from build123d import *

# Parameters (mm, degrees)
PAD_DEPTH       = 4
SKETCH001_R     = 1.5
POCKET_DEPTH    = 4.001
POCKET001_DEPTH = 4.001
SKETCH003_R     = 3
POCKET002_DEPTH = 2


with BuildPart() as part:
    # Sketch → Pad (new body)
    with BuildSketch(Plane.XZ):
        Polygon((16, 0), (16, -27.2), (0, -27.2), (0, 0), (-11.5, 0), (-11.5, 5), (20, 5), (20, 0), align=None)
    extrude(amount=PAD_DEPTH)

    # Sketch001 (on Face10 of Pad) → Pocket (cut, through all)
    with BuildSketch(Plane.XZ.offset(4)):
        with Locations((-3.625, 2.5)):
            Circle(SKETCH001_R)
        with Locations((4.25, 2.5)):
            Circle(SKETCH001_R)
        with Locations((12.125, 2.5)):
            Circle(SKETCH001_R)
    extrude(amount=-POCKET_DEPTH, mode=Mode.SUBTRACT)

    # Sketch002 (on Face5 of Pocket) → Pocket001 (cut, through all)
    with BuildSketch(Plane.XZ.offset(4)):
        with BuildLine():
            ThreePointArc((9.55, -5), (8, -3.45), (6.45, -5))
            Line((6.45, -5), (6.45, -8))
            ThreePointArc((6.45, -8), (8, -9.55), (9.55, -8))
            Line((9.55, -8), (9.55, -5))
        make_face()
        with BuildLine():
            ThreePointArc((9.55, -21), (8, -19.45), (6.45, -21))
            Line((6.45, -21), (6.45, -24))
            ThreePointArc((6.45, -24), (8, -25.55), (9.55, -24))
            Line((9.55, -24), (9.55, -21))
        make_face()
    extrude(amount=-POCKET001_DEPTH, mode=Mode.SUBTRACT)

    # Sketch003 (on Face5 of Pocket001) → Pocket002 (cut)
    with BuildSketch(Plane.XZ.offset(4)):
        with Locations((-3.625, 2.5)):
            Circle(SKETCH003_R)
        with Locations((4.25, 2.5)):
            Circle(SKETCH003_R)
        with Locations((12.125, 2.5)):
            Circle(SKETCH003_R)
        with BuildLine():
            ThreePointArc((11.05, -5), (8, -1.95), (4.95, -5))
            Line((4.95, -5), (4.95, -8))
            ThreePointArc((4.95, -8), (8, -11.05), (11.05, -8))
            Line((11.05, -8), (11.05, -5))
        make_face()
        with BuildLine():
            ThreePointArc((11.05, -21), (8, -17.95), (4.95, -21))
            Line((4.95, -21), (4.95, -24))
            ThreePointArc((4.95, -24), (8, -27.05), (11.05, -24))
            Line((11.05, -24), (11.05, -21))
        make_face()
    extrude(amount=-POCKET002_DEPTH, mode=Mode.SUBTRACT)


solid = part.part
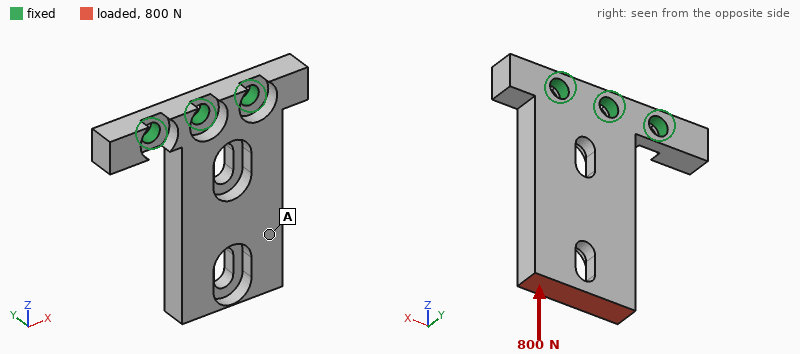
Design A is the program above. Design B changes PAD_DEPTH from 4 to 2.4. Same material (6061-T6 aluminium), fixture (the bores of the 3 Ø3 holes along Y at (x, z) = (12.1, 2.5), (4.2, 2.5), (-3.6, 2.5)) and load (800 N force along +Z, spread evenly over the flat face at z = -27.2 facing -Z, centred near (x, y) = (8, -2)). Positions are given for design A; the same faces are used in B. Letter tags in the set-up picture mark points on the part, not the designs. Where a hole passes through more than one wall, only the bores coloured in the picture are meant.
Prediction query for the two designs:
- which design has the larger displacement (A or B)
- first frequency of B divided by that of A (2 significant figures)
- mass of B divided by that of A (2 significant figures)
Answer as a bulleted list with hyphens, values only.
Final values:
- A
- 0.76
- 0.65
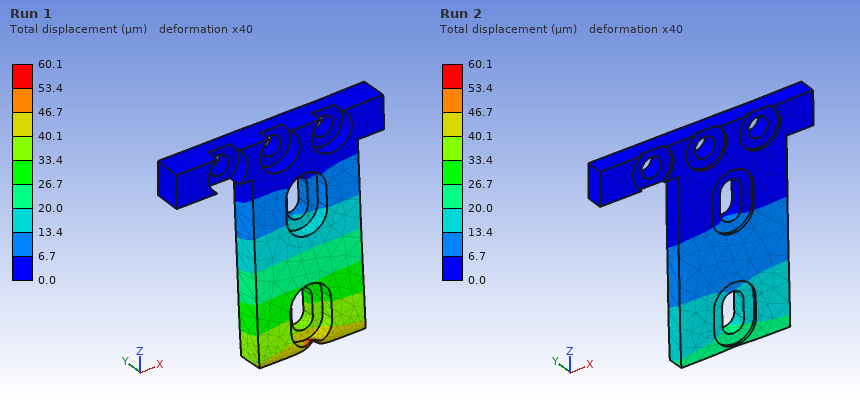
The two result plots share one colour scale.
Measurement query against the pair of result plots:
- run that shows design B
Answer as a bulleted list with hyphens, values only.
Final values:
- Run 2
